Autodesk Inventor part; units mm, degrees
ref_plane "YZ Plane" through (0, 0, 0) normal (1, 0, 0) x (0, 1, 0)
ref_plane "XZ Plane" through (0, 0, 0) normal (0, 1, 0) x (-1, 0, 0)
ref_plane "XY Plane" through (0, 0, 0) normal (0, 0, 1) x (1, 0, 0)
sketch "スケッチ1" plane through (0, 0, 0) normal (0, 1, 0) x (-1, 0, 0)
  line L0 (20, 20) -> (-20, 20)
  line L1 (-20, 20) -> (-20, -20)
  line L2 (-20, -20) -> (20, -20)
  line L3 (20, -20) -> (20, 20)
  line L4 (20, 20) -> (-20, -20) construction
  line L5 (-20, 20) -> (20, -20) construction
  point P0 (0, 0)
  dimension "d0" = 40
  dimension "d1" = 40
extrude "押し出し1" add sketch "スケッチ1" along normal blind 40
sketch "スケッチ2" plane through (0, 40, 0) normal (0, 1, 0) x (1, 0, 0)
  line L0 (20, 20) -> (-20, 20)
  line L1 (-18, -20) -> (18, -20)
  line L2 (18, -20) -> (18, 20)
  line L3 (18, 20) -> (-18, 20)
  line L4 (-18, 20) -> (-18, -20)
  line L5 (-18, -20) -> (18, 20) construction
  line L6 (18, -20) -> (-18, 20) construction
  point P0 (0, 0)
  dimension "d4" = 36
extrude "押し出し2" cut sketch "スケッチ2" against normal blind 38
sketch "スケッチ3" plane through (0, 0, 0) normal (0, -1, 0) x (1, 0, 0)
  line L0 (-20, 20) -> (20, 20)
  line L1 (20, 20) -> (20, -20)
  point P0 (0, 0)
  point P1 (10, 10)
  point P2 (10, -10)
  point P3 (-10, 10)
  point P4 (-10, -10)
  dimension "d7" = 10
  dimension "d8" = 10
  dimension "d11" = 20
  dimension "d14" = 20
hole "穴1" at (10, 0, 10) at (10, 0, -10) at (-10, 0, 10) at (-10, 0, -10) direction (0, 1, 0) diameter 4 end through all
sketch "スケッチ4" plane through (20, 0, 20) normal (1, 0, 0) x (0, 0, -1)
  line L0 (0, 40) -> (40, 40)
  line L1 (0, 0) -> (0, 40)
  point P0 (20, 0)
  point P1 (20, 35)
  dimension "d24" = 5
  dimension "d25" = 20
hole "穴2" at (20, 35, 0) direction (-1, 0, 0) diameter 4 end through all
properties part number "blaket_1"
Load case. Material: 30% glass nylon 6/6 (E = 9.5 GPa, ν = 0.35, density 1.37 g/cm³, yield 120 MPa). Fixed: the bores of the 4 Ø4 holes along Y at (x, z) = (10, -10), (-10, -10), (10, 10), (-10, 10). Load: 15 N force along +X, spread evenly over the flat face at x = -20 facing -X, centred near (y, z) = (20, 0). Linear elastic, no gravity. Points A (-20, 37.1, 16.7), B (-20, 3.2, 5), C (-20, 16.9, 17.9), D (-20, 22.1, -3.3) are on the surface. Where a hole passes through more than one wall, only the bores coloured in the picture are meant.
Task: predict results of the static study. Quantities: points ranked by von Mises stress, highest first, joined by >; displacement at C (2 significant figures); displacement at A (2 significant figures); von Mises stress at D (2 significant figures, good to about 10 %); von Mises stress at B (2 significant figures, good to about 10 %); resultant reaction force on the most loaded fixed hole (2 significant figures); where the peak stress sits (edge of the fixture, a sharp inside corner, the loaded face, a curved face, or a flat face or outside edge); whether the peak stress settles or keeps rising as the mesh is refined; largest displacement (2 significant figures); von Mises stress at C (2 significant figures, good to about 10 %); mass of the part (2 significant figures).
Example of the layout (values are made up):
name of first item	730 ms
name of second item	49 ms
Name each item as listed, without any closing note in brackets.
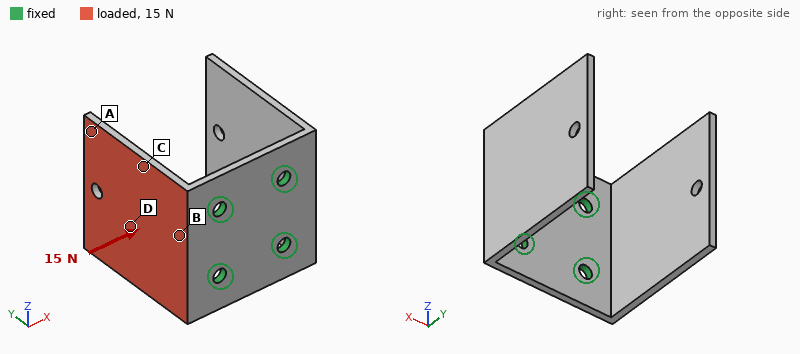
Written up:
points ranked by von Mises stress, highest first, joined by >	B > C > D > A
displacement at C	0.23 mm
displacement at A	0.64 mm
von Mises stress at D	2.0 MPa
von Mises stress at B	8.7 MPa
resultant reaction force on the most loaded fixed hole	6.8 N
where the peak stress sits	edge of the fixture
whether the peak stress settles or keeps rising as the mesh is refined	keeps rising
largest displacement	0.71 mm
von Mises stress at C	3.8 MPa
mass of the part	13 g
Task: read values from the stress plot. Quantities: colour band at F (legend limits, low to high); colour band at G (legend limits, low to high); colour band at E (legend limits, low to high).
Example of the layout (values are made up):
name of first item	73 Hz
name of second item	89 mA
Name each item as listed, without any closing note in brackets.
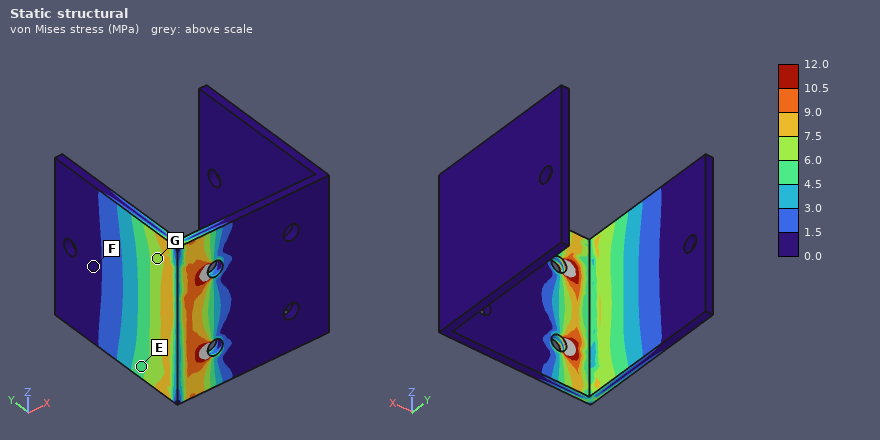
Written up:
colour band at F	0.0 to 1.5 MPa
colour band at G	6.0 to 7.5 MPa
colour band at E	4.5 to 6.0 MPa
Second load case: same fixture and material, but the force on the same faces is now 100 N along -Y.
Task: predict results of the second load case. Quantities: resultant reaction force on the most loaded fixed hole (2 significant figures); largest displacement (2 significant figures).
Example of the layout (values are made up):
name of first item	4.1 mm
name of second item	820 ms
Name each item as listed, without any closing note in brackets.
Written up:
resultant reaction force on the most loaded fixed hole	54 N
largest displacement	0.83 mm
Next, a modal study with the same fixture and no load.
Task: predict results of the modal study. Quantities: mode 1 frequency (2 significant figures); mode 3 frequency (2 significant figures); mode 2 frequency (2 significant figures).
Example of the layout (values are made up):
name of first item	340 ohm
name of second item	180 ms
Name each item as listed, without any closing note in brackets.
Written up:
mode 1 frequency	440 Hz
mode 3 frequency	1100 Hz
mode 2 frequency	440 Hz
